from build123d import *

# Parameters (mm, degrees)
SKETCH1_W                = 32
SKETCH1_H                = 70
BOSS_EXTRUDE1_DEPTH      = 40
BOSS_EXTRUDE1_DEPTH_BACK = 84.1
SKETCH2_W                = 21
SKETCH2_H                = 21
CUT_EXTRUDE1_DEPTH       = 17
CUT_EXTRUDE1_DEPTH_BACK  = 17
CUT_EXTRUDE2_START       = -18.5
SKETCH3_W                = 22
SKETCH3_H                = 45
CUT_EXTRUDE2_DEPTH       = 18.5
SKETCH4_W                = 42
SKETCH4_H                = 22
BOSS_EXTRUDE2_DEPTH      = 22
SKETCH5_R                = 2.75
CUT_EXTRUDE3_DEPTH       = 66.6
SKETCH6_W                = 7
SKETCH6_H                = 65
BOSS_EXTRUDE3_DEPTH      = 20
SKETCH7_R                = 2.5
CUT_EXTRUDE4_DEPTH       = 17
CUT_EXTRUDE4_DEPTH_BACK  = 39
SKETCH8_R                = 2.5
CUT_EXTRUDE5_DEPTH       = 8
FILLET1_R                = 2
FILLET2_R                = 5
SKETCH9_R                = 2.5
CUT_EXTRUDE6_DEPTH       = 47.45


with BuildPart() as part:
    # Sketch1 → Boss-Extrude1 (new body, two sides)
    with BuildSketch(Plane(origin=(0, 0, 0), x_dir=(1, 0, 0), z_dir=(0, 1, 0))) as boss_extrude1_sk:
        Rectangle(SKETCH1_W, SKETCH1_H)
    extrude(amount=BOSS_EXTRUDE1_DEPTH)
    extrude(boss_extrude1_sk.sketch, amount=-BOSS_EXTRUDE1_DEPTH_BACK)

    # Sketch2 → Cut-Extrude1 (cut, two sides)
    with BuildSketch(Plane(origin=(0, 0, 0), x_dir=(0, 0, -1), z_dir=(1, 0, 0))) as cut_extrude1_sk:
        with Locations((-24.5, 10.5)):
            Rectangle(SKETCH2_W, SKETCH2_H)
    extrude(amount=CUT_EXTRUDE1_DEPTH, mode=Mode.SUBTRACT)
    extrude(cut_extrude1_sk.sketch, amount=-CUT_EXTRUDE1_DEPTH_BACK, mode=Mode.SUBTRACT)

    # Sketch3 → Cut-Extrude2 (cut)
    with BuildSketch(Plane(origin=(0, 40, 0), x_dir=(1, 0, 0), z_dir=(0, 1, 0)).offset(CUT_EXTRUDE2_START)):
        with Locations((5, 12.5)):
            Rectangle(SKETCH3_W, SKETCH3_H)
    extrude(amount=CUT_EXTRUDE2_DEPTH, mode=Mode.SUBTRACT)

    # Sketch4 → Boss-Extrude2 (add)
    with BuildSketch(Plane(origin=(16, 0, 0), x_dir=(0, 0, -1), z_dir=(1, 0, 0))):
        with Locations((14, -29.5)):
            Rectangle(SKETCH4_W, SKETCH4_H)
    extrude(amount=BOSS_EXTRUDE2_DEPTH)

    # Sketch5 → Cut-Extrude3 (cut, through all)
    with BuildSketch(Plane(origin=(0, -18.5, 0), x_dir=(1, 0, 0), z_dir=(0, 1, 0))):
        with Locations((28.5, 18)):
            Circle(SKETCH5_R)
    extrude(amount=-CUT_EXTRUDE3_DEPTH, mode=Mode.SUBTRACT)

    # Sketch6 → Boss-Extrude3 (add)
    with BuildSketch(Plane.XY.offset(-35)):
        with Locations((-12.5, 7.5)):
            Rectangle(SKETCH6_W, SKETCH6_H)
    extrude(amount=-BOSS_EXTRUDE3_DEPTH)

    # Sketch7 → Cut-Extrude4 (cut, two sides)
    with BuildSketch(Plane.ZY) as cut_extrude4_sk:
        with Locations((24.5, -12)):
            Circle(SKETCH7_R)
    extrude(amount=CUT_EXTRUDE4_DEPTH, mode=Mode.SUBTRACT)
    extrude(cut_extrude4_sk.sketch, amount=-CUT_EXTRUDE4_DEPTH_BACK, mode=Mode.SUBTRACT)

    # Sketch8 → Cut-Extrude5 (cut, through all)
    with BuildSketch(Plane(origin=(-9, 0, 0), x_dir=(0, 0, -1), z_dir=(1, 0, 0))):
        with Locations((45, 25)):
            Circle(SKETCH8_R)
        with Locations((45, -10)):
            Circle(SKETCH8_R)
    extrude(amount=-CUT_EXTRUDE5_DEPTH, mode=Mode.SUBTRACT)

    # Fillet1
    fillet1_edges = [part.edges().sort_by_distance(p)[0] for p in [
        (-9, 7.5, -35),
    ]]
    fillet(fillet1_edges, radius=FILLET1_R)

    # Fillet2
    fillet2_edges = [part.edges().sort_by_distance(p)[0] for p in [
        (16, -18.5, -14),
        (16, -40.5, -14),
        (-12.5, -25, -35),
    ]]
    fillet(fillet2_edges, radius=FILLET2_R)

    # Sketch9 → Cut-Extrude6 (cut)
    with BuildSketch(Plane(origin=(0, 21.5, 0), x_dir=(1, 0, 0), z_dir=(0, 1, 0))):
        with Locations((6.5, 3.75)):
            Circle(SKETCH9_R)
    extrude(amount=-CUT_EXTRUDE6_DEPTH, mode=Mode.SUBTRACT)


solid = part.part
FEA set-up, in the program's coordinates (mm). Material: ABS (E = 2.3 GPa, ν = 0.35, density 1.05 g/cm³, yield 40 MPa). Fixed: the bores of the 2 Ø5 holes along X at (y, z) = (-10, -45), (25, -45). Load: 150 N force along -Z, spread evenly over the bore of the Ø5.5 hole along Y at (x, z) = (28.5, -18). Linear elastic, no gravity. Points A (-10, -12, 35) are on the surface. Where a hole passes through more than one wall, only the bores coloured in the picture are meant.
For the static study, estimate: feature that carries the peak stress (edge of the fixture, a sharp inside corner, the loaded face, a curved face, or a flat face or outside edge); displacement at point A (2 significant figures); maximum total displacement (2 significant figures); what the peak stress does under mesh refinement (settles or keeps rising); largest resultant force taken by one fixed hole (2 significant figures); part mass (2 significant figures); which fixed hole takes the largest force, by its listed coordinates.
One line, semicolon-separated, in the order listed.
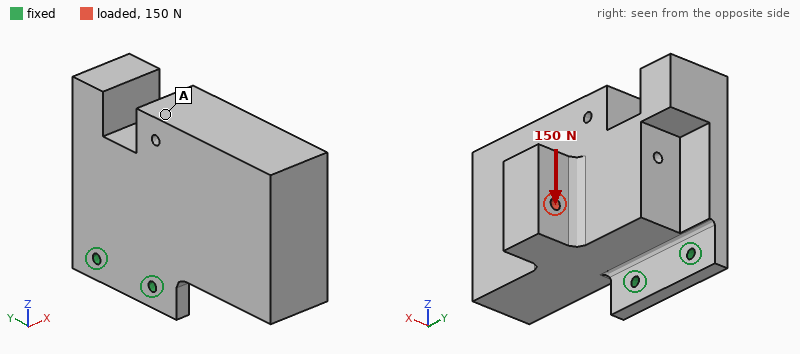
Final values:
edge of the fixture; 1.6 mm; 1.8 mm; keeps rising; 220 N; 290 g; (-10, -45)
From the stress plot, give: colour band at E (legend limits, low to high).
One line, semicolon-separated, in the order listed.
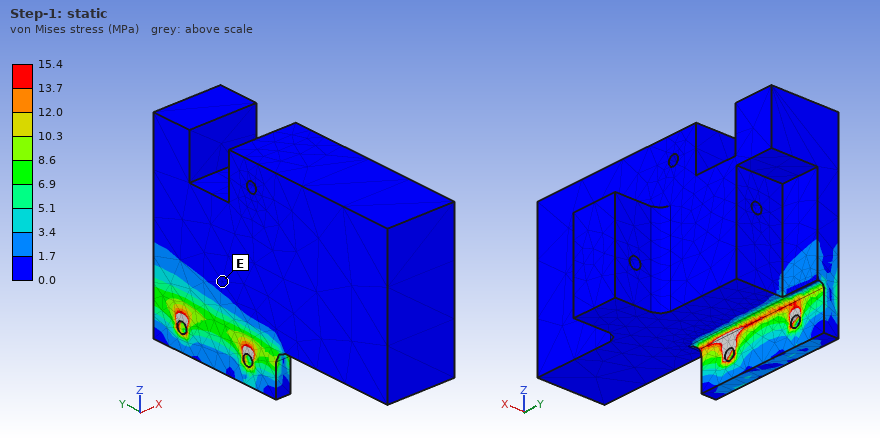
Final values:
0.0 to 1.7 MPa
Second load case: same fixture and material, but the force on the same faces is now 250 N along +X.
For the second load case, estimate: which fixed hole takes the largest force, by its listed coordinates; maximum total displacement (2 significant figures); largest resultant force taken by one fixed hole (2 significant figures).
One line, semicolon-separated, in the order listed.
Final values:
(-10, -45); 1.9 mm; 360 N
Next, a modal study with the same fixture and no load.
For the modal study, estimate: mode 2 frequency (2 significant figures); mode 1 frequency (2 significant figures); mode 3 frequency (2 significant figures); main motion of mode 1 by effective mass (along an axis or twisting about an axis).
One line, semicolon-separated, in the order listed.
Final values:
330 Hz; 110 Hz; 440 Hz; along X
